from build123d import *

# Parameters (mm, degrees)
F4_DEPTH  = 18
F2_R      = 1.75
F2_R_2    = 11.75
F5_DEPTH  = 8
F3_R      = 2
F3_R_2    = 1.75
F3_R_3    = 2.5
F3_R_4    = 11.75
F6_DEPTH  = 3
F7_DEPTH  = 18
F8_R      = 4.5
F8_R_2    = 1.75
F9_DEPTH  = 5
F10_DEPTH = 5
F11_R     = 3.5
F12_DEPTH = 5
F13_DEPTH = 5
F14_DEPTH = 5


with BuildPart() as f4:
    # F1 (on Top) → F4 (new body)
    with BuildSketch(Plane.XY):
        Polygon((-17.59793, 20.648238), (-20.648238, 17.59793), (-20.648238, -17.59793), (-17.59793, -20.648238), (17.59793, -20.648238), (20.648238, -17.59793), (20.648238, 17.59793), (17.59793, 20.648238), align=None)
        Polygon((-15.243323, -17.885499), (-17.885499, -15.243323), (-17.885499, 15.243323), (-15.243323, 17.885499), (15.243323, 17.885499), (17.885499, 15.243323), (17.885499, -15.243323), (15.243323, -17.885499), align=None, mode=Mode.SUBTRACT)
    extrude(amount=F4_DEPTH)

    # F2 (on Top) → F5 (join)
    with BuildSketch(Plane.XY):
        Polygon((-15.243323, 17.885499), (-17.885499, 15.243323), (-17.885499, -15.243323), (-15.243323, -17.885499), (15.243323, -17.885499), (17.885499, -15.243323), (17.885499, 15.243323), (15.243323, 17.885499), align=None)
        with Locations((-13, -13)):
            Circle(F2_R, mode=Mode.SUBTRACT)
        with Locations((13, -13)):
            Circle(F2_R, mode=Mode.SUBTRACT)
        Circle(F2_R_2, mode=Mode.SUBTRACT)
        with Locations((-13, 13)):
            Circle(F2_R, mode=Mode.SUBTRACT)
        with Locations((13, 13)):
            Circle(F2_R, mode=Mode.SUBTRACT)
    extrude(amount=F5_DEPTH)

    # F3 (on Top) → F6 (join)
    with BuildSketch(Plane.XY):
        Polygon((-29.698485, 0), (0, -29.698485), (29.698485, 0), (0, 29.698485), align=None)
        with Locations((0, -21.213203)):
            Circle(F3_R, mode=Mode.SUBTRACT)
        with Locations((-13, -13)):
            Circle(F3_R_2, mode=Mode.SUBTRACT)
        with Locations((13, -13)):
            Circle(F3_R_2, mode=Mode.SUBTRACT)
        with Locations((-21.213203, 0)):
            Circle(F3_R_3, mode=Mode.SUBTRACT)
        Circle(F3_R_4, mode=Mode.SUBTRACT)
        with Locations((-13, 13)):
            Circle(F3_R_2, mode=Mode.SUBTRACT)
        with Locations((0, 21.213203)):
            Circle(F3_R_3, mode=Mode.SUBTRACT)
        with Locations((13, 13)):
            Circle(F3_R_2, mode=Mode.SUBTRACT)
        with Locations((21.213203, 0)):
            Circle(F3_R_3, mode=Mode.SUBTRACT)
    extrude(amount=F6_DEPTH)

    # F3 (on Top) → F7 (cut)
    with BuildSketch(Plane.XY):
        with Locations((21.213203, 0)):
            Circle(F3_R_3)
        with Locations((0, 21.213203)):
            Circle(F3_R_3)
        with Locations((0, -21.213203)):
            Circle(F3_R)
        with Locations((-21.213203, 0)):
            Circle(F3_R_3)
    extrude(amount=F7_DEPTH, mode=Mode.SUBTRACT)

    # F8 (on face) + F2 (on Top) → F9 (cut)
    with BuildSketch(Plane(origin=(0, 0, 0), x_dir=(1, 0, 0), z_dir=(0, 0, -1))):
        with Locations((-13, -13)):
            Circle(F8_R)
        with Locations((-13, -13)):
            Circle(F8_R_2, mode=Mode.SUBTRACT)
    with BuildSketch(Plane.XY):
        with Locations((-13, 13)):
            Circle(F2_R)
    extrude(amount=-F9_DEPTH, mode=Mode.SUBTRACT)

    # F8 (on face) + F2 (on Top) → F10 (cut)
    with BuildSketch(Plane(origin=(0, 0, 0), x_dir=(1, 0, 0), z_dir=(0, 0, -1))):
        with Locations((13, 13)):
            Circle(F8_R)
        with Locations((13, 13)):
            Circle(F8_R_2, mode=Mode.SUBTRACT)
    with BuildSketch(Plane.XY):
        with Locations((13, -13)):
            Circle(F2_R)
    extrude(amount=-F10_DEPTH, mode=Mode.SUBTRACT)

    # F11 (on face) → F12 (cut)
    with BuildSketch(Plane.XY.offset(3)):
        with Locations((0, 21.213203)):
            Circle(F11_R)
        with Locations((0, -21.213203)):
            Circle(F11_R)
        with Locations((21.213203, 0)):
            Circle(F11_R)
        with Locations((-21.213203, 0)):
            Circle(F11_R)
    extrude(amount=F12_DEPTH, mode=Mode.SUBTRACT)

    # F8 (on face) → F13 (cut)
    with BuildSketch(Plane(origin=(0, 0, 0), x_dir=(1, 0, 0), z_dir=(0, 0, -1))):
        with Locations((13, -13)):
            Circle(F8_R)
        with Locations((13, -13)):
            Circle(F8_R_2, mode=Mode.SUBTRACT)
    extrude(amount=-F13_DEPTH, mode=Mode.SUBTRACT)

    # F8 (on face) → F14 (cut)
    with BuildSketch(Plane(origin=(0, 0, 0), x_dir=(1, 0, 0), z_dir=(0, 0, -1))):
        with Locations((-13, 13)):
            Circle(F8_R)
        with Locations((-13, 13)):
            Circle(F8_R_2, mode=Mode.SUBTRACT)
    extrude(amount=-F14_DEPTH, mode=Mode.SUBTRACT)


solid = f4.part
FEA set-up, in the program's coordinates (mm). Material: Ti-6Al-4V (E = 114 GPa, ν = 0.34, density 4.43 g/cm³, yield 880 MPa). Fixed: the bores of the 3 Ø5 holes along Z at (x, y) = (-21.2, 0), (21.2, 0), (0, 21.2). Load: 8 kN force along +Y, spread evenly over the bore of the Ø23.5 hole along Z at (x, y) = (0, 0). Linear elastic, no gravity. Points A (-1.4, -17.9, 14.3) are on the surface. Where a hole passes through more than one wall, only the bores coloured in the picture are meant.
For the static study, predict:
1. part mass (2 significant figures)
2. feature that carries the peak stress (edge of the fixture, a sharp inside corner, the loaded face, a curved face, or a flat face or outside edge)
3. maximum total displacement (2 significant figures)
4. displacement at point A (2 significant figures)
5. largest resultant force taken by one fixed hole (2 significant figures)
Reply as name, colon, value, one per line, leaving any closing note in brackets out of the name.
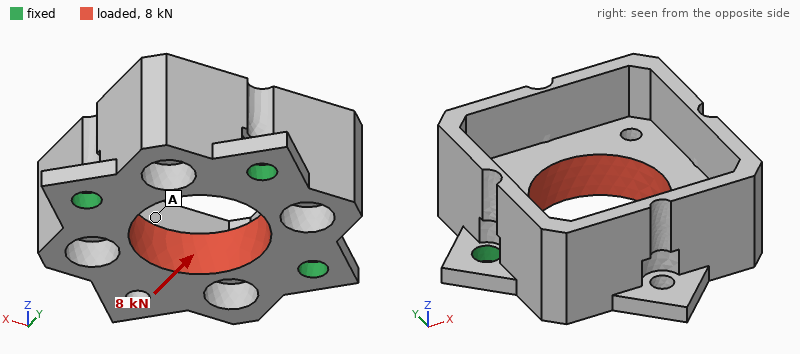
part mass: 58 g
feature that carries the peak stress: edge of the fixture
maximum total displacement: 26 µm
displacement at point A: 24 µm
largest resultant force taken by one fixed hole: 2.9 kN
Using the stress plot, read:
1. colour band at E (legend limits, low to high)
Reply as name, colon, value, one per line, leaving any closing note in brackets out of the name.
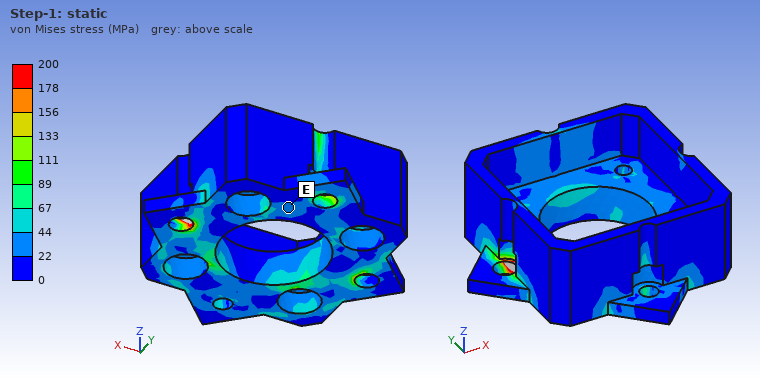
colour band at E: 22 to 44 MPa
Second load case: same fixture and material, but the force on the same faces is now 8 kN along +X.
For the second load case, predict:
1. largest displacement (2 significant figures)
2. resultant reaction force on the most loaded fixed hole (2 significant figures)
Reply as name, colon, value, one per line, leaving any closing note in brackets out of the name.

largest displacement: 17 µm
resultant reaction force on the most loaded fixed hole: 3.3 kN
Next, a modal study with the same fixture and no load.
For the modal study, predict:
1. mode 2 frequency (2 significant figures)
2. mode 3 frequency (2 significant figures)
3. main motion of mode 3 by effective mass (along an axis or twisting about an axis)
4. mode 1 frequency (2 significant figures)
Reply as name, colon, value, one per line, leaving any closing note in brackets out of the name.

mode 2 frequency: 9800 Hz
mode 3 frequency: 15 kHz
main motion of mode 3 by effective mass: along X
mode 1 frequency: 6600 Hz
